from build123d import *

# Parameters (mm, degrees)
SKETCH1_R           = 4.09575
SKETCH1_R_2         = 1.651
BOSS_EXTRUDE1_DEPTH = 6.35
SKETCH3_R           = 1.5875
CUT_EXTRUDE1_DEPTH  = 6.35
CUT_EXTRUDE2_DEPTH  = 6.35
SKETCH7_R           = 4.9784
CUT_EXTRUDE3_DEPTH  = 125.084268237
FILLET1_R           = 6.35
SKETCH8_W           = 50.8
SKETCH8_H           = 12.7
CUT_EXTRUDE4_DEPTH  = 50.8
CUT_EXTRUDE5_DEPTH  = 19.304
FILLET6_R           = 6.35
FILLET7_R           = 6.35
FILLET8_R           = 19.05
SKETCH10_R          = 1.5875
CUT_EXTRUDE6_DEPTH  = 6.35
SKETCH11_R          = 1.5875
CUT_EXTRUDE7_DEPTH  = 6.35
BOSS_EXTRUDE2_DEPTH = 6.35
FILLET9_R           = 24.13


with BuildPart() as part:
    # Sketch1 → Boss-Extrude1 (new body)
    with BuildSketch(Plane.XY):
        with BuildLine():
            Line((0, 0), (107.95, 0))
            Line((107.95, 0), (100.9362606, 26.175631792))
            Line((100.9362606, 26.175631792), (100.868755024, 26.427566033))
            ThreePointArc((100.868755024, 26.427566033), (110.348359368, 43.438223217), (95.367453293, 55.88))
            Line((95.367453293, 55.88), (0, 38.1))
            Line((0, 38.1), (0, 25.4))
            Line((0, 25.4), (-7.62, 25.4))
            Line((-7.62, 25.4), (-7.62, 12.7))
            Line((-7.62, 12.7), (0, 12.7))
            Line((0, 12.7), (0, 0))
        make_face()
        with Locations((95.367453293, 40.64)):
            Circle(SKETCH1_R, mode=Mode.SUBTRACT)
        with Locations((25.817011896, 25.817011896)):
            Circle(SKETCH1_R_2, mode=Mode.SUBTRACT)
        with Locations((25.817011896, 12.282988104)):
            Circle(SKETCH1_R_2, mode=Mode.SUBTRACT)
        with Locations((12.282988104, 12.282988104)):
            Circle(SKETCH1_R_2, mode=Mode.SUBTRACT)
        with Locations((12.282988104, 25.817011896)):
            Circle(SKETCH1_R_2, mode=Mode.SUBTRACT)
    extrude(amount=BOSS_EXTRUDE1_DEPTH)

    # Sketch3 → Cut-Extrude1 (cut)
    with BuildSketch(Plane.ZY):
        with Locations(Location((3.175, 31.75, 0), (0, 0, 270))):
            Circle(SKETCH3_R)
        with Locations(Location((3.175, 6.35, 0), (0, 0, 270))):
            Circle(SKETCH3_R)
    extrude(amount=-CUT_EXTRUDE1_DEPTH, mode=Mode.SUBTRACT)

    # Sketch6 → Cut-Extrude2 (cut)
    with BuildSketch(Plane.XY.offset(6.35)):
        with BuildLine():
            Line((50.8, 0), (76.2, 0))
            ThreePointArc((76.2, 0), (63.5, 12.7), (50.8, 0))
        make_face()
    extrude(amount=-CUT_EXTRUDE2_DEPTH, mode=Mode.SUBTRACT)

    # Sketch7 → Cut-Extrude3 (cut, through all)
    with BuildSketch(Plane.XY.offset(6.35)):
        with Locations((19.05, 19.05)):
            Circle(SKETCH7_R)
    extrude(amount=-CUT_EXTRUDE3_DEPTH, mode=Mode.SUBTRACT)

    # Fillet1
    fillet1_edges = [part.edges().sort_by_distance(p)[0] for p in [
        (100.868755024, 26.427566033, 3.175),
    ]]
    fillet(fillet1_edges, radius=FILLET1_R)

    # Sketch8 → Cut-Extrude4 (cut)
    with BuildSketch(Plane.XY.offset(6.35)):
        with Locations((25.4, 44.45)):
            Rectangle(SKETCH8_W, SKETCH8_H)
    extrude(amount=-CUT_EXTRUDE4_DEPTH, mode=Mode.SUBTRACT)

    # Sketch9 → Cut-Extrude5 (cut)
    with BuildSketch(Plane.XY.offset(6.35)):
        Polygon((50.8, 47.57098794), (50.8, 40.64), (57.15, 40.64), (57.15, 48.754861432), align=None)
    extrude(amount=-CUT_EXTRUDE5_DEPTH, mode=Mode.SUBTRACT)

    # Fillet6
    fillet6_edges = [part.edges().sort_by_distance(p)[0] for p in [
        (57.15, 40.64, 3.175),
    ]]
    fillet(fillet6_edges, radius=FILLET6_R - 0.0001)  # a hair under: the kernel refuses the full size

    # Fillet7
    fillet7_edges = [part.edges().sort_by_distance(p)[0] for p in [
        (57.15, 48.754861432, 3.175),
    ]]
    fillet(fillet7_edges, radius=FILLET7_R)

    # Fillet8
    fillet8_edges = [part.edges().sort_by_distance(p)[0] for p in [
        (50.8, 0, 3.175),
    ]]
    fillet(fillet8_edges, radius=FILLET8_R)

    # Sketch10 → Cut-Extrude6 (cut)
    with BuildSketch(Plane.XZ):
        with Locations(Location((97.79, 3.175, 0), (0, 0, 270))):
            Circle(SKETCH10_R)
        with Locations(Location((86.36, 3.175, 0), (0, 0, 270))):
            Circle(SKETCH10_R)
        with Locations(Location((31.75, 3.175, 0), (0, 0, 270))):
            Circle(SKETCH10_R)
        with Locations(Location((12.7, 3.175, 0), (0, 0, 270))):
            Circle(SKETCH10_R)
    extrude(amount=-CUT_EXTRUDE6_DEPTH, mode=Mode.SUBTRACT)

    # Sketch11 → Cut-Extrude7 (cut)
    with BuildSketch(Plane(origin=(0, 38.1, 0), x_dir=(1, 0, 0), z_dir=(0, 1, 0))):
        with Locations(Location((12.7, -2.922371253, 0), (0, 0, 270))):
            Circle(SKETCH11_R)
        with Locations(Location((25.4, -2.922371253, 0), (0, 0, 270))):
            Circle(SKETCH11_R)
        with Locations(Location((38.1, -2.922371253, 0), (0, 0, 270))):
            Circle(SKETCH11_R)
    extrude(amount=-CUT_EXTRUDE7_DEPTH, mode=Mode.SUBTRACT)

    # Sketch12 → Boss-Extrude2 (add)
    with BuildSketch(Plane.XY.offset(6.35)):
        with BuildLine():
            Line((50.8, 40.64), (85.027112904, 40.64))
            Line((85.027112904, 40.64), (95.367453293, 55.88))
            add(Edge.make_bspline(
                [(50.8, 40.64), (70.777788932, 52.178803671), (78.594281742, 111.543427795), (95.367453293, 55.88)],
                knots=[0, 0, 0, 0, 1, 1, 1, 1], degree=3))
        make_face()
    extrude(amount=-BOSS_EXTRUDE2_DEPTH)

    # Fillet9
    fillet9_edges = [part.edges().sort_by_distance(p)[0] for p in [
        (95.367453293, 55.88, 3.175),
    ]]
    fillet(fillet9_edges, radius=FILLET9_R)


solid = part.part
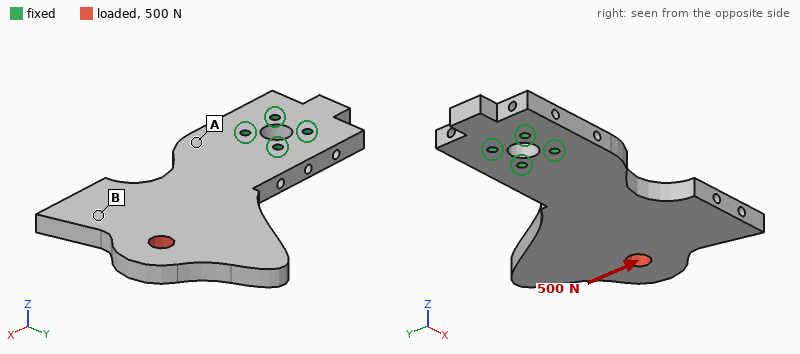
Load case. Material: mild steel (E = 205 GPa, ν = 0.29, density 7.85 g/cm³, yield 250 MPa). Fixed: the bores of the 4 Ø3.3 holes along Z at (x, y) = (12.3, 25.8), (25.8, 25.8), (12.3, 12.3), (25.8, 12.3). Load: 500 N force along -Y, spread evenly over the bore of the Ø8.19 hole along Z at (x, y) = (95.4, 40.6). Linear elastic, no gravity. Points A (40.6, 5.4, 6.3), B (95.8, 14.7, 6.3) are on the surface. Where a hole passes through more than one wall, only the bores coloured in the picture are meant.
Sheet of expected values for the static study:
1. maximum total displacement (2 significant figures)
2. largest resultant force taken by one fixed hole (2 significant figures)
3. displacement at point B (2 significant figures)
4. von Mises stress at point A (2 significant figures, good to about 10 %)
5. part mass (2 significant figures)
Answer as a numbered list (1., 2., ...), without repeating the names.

1. 27 µm
2. 1.4 kN
3. 21 µm
4. 14 MPa
5. 250 g
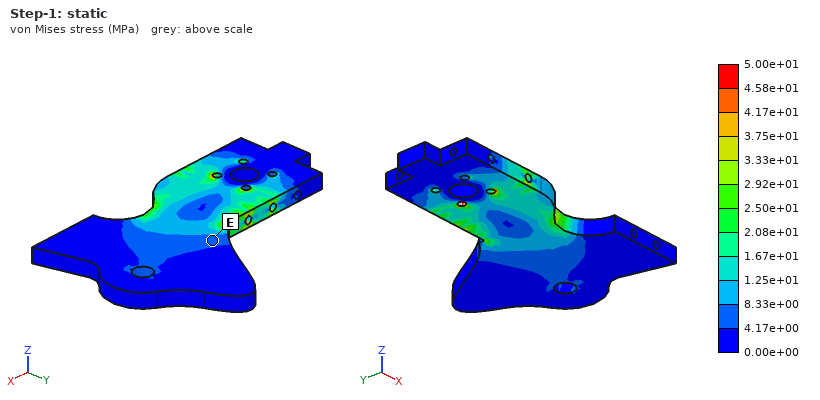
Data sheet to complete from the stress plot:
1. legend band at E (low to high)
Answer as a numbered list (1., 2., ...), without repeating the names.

1. 4.17e+00 to 8.33e+00 MPa
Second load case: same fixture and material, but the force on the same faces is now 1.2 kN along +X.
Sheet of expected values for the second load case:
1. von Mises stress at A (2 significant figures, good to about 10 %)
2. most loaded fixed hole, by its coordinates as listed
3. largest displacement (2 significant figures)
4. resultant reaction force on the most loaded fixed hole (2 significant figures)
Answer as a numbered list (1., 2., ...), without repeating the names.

1. 8.0 MPa
2. (25.8, 25.8)
3. 22 µm
4. 1.5 kN
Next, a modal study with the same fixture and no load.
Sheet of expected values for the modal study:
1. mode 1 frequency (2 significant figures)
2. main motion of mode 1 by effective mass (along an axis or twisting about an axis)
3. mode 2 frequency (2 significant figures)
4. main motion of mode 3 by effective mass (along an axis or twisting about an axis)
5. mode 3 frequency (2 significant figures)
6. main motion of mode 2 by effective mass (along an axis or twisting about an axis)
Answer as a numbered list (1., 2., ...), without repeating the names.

1. 580 Hz
2. along Z
3. 1400 Hz
4. along Y
5. 2300 Hz
6. twisting about X
